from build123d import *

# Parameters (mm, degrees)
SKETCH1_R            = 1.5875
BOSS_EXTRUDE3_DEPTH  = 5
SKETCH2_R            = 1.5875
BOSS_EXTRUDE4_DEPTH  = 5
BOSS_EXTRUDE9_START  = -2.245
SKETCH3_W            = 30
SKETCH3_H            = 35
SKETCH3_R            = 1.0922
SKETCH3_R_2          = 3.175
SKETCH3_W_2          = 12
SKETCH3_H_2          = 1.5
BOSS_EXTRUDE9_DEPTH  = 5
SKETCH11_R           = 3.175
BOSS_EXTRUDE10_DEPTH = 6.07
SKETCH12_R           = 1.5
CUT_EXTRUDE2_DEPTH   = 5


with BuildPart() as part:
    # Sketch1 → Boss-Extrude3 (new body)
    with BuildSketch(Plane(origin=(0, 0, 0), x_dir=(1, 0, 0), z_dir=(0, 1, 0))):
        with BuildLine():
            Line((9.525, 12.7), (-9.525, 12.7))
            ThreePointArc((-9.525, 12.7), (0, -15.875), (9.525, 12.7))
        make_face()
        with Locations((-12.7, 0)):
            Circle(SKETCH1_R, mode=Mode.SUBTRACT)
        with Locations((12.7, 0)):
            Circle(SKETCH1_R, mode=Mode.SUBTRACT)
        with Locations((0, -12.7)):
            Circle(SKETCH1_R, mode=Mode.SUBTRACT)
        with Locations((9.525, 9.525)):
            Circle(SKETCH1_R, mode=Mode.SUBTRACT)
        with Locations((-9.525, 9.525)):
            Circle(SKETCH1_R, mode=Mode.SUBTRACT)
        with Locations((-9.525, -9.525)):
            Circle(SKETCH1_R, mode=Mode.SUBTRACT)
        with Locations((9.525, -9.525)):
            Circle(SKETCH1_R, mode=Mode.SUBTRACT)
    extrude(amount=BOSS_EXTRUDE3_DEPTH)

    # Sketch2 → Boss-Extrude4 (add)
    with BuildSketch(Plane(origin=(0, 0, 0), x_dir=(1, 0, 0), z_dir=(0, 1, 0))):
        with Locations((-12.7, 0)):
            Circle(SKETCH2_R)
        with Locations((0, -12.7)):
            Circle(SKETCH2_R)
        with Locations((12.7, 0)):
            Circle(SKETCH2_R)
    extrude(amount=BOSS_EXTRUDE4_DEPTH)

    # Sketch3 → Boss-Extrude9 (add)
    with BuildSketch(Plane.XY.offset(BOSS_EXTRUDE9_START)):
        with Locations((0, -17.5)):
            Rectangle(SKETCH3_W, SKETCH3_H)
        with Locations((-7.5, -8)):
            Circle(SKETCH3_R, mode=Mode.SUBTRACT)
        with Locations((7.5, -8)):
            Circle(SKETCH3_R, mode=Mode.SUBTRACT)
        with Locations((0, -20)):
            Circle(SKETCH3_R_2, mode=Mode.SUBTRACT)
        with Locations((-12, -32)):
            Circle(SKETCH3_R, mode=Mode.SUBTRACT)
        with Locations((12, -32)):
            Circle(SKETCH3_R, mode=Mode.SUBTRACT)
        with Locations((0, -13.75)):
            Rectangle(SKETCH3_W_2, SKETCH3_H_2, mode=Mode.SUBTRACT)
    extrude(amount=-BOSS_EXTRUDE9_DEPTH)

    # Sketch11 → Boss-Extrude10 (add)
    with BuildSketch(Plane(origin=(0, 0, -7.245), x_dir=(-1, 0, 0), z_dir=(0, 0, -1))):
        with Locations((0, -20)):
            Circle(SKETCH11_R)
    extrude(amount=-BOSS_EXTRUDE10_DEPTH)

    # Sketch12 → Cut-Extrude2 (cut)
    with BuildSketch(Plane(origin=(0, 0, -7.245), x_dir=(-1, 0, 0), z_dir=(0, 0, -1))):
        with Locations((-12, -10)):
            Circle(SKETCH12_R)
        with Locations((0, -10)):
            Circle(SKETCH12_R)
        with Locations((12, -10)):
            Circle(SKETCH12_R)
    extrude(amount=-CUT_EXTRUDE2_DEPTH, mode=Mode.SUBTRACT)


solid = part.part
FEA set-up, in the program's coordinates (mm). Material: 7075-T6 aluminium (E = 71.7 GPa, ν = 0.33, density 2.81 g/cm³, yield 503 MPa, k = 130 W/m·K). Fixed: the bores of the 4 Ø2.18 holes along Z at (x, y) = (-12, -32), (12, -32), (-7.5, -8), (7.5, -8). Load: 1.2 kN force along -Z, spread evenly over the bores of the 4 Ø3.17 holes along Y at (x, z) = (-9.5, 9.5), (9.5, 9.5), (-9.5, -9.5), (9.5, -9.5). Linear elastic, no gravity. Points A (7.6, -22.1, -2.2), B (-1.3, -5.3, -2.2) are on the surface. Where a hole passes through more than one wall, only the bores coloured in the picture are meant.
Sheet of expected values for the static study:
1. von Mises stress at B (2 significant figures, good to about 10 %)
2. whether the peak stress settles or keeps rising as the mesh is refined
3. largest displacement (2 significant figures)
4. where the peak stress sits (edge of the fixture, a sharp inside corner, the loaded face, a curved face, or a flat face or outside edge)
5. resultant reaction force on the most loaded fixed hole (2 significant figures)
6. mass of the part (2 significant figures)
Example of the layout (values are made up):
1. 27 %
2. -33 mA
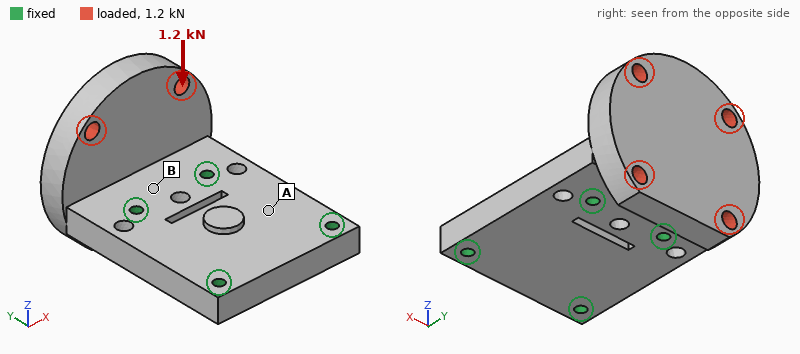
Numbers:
1. 44 MPa
2. keeps rising
3. 90 µm
4. edge of the fixture
5. 650 N
6. 24 g
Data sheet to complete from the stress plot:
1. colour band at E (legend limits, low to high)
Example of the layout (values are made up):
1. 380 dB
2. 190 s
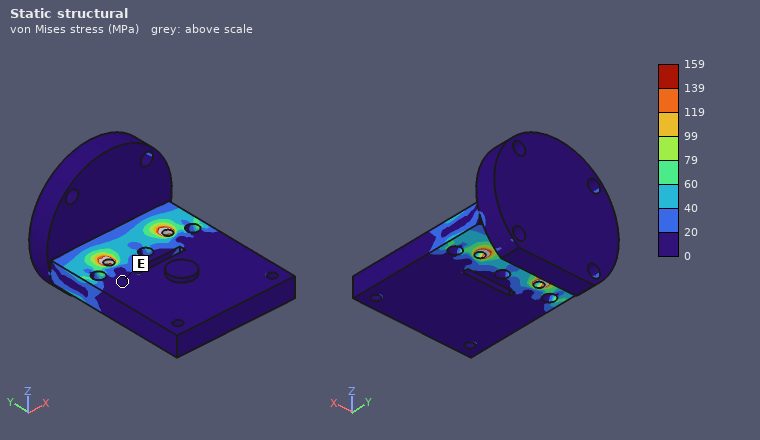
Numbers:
1. 0 to 20 MPa
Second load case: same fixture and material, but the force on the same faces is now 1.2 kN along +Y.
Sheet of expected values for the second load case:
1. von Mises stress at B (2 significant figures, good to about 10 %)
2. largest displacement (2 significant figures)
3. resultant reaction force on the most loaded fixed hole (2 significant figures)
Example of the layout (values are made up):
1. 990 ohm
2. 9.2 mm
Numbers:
1. 34 MPa
2. 96 µm
3. 560 N
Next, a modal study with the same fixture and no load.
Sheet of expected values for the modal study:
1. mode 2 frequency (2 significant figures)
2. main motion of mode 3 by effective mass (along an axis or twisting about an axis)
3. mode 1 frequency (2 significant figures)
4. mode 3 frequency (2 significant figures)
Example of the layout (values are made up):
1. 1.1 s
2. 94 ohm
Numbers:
1. 11 kHz
2. along Z
3. 5800 Hz
4. 16 kHz
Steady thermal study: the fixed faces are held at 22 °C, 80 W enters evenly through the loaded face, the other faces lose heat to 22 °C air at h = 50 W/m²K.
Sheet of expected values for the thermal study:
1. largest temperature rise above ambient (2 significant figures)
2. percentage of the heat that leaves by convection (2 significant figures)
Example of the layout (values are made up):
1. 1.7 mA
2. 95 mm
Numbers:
1. 76 K
2. 7.3 %
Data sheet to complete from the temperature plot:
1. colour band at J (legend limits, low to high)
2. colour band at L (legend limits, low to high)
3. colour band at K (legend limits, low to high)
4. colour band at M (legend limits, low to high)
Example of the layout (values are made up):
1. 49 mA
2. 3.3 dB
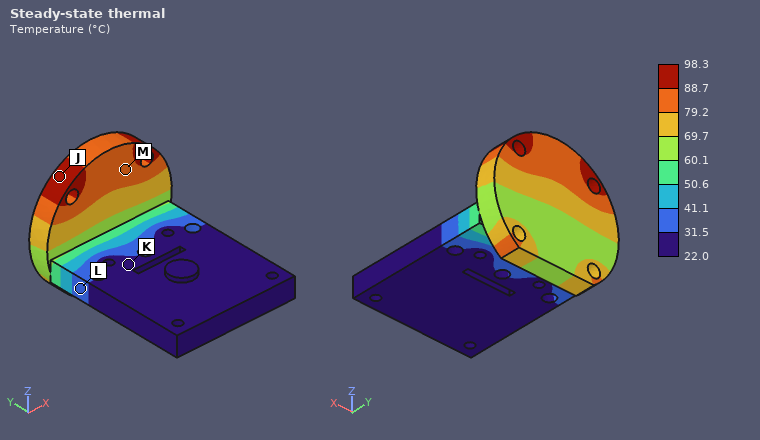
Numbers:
1. 88.7 to 98.3 °C
2. 31.5 to 41.1 °C
3. 22.0 to 31.5 °C
4. 79.2 to 88.7 °C
